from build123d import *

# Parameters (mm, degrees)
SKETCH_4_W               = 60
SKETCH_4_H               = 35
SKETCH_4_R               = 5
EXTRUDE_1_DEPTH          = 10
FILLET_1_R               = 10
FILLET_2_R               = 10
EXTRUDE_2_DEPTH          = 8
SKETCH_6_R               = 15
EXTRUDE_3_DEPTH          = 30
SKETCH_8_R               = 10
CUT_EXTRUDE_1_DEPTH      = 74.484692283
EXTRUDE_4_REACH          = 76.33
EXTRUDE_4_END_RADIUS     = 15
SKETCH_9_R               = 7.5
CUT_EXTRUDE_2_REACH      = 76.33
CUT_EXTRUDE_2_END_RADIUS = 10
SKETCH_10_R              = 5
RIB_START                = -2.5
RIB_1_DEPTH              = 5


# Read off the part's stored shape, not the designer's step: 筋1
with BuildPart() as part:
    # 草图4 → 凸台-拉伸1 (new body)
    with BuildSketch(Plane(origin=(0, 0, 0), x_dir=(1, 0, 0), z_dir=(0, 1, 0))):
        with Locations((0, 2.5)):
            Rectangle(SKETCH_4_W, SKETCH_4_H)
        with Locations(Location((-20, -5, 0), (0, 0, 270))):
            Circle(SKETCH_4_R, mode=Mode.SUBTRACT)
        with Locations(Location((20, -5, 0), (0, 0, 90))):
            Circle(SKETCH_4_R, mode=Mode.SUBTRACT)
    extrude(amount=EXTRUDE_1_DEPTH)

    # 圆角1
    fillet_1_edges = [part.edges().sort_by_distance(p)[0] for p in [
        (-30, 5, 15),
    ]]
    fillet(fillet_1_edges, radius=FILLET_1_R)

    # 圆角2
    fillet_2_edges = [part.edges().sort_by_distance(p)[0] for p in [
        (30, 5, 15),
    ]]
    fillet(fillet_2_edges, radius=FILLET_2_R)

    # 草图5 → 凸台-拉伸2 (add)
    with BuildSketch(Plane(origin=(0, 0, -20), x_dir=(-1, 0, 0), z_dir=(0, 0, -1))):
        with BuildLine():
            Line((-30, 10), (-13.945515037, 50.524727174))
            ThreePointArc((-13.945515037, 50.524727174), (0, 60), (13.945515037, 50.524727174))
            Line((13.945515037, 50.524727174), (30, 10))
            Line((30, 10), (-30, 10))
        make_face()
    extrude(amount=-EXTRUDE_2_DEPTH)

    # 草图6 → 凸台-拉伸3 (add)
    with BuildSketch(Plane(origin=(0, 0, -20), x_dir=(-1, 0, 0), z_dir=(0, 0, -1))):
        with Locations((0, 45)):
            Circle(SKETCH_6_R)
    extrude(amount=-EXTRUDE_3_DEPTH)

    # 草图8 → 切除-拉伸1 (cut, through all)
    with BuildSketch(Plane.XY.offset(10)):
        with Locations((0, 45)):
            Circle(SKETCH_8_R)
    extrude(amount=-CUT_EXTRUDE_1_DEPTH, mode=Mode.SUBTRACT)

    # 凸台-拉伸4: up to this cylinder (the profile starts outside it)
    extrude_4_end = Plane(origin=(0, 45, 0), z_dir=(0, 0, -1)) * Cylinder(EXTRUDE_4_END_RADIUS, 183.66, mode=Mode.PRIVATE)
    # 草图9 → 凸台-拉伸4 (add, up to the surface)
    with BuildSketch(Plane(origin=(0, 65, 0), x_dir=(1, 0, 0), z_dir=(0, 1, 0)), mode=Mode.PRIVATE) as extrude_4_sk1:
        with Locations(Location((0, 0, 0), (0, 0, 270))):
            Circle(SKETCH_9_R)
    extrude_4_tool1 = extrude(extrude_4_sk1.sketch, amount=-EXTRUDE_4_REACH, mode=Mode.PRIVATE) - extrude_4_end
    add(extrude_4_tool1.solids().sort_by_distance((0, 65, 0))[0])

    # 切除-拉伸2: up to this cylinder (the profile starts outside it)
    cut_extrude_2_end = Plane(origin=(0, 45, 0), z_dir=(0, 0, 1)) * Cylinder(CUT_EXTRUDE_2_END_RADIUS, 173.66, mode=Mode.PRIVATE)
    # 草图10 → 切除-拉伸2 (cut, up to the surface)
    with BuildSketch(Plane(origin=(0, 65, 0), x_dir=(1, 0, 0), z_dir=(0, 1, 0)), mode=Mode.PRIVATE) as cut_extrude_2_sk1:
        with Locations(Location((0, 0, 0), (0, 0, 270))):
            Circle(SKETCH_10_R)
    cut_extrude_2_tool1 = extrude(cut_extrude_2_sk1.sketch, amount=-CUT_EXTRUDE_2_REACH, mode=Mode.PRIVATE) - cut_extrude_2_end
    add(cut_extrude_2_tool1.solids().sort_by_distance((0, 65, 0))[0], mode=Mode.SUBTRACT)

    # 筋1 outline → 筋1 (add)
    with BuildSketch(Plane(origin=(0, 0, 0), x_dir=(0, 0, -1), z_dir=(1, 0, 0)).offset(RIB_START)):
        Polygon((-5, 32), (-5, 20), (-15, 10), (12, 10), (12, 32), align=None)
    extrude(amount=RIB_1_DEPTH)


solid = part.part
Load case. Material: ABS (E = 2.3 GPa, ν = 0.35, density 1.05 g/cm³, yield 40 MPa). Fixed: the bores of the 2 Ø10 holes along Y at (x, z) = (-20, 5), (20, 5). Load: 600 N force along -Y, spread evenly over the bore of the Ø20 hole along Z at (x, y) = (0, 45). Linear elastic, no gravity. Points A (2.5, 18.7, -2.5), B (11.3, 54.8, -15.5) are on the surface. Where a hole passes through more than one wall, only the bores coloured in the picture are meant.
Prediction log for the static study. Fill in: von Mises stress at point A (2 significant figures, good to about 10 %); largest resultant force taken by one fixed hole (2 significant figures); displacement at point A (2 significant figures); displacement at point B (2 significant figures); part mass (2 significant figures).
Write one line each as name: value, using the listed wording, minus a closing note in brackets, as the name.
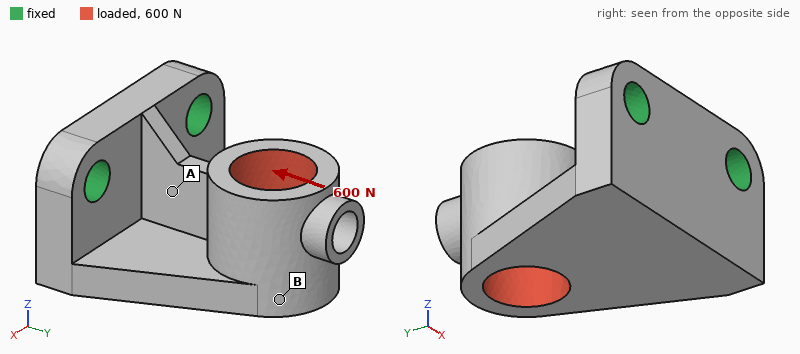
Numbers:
von Mises stress at point A: 4.1 MPa
largest resultant force taken by one fixed hole: 300 N
displacement at point A: 0.068 mm
displacement at point B: 0.093 mm
part mass: 45 g
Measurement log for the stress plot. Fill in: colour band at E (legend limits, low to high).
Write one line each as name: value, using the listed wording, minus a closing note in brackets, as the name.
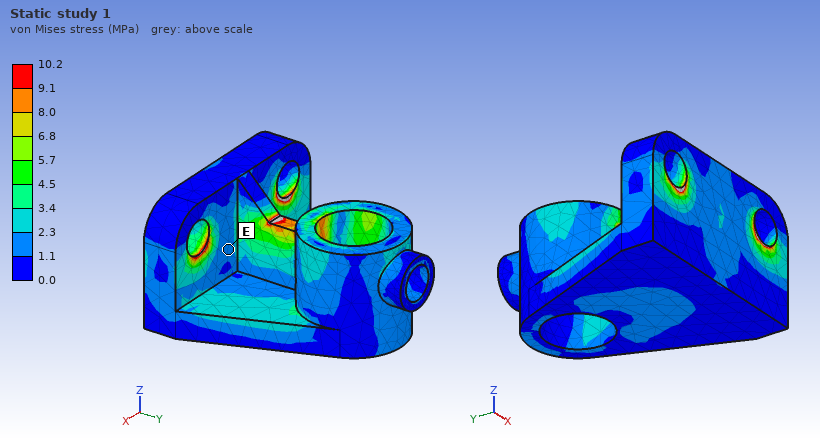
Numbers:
colour band at E: 1.1 to 2.3 MPa
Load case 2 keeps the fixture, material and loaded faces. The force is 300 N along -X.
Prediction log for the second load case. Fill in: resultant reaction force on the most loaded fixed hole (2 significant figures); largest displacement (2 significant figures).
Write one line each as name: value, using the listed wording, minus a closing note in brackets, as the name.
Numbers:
resultant reaction force on the most loaded fixed hole: 330 N
largest displacement: 0.57 mm
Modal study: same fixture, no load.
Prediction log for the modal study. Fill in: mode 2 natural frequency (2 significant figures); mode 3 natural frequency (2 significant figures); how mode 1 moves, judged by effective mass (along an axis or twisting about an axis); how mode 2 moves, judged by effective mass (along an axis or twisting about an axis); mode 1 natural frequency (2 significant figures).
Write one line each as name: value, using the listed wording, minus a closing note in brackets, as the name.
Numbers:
mode 2 natural frequency: 1100 Hz
mode 3 natural frequency: 2300 Hz
how mode 1 moves, judged by effective mass: along Z
how mode 2 moves, judged by effective mass: along X
mode 1 natural frequency: 890 Hz
